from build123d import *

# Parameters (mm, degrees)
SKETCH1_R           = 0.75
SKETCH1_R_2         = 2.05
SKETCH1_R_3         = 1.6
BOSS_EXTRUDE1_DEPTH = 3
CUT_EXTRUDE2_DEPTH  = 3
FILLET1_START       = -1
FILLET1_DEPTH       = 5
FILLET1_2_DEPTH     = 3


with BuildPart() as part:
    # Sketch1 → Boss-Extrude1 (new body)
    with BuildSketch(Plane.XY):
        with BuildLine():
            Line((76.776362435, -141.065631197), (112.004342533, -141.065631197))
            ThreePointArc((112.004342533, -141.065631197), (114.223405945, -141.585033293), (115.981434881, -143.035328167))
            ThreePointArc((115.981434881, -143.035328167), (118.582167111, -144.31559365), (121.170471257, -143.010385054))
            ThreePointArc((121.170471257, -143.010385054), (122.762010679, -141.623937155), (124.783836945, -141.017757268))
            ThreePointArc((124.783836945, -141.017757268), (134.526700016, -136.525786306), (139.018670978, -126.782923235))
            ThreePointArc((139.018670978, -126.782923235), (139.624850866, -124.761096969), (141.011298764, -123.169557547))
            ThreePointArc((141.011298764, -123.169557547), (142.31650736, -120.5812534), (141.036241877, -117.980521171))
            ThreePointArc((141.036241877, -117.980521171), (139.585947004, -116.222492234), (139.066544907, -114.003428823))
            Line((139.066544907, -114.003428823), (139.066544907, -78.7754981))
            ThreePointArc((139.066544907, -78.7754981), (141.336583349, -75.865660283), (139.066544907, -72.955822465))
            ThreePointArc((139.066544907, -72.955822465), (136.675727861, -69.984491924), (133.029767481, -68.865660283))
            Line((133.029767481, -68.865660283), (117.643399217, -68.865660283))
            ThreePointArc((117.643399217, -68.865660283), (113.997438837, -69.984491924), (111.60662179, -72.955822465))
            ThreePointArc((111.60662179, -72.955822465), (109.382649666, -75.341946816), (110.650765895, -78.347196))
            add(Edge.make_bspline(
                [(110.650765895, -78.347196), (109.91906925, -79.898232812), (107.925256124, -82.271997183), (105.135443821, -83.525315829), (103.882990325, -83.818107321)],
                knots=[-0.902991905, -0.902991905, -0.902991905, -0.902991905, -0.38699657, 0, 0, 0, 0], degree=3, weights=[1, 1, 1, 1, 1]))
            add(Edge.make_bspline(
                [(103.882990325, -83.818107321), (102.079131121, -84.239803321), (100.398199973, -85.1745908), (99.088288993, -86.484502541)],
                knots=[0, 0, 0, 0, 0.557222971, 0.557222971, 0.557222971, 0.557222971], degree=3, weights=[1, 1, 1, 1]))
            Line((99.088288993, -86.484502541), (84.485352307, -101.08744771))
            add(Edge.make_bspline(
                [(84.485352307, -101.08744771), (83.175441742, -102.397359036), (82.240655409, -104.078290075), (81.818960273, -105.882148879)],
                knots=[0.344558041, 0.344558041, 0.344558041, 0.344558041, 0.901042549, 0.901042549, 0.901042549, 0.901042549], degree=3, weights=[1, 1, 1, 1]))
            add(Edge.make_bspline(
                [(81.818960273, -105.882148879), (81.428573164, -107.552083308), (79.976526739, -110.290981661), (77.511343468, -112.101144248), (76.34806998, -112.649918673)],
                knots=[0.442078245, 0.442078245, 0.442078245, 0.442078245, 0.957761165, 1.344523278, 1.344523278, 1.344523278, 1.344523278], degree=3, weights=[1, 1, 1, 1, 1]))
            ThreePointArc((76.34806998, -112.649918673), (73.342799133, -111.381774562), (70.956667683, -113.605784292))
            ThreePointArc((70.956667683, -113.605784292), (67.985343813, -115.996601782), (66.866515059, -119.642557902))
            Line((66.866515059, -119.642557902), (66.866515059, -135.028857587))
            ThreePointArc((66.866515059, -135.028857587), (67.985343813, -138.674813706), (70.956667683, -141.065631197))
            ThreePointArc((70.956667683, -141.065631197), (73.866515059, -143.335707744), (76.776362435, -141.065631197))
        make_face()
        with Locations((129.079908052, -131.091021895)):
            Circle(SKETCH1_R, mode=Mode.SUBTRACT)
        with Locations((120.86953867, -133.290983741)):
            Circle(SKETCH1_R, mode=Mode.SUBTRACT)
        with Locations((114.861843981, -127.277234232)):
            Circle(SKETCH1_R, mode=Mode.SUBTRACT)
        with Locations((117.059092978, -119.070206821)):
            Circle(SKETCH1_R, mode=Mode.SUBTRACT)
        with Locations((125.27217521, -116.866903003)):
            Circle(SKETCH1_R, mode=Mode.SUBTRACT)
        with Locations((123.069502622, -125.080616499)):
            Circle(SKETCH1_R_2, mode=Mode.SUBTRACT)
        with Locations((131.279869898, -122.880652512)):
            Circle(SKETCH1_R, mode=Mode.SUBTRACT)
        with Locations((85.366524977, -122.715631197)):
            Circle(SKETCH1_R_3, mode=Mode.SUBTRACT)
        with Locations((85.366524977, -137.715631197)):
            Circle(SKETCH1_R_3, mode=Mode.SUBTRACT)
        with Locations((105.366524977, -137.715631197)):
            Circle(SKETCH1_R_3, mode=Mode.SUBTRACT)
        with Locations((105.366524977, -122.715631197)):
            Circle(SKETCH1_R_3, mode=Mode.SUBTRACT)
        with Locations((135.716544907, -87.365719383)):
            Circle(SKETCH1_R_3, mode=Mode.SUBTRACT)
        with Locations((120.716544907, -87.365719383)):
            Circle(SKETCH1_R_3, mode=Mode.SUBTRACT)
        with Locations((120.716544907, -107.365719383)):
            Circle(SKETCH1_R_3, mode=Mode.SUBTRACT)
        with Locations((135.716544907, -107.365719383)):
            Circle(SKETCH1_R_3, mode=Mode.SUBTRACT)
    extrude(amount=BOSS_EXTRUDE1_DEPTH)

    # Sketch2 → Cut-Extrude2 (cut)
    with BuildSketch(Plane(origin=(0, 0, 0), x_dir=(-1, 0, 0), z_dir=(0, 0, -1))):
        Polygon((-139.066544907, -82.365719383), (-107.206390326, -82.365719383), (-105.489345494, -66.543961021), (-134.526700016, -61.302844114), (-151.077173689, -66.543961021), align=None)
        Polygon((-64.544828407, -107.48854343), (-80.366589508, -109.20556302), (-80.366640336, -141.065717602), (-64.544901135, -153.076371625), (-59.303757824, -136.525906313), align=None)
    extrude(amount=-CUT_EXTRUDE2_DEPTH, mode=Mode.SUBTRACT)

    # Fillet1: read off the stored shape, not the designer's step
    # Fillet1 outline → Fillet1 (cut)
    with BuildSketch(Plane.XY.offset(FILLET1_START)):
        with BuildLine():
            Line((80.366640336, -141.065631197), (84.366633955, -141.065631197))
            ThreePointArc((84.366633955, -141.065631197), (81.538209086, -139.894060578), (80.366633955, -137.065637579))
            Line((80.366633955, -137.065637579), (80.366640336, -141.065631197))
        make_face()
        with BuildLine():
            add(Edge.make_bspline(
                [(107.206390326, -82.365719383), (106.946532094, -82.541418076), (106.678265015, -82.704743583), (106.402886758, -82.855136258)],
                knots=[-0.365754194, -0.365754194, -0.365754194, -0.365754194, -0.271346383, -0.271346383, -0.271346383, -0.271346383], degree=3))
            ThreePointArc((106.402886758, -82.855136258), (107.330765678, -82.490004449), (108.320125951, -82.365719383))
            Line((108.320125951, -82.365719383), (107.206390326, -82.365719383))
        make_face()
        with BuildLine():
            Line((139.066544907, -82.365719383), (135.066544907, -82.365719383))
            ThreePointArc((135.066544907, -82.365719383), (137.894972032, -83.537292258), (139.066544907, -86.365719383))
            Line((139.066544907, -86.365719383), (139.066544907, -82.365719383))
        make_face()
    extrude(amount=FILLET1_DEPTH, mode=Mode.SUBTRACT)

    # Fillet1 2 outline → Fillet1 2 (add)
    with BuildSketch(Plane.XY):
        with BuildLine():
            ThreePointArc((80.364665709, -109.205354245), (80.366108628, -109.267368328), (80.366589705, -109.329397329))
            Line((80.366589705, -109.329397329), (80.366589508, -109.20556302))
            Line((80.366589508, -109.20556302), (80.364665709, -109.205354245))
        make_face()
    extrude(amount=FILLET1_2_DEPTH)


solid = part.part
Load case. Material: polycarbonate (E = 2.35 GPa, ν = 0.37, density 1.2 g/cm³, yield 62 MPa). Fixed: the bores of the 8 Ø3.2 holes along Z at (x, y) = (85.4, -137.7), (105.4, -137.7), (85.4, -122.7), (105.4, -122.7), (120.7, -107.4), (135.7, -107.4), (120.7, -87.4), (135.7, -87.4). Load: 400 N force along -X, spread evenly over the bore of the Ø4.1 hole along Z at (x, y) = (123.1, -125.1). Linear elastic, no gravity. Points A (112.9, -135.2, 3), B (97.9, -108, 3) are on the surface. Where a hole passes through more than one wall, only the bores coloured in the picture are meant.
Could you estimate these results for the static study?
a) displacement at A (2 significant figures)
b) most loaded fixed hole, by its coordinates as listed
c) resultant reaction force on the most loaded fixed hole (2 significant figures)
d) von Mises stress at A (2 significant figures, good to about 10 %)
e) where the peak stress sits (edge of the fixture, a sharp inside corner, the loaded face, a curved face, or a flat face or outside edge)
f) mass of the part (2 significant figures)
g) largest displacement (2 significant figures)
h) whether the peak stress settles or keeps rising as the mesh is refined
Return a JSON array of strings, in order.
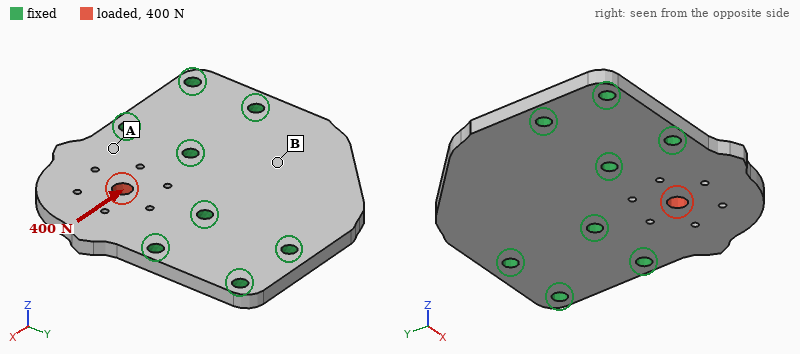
["14 µm", "(105.4, -122.7)", "150 N", "3.9 MPa", "a sharp inside corner", "11 g", "56 µm", "keeps rising"]
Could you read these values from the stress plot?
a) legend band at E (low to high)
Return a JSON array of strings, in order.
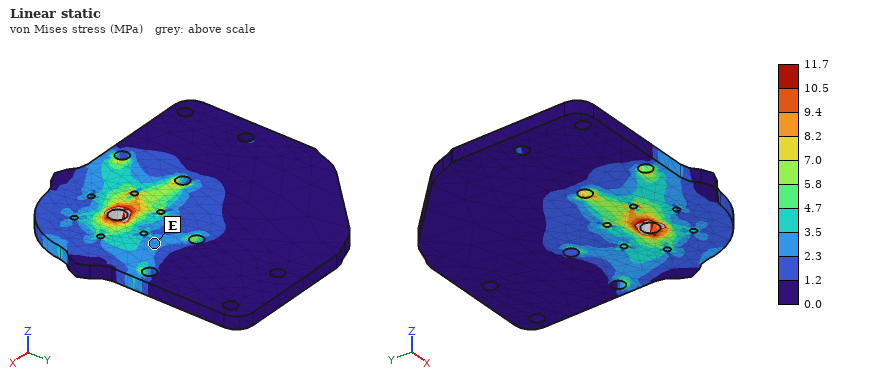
["2.3 to 3.5 MPa"]
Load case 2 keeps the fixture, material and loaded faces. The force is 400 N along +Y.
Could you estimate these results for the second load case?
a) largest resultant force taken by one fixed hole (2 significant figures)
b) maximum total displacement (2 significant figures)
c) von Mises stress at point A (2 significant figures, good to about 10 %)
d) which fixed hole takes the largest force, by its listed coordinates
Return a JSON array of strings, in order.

["150 N", "57 µm", "3.3 MPa", "(120.7, -107.4)"]
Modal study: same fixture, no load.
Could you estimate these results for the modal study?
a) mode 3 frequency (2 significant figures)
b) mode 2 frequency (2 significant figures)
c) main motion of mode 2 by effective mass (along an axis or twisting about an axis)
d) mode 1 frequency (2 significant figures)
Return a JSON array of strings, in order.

["3500 Hz", "1500 Hz", "along Z", "1400 Hz"]
